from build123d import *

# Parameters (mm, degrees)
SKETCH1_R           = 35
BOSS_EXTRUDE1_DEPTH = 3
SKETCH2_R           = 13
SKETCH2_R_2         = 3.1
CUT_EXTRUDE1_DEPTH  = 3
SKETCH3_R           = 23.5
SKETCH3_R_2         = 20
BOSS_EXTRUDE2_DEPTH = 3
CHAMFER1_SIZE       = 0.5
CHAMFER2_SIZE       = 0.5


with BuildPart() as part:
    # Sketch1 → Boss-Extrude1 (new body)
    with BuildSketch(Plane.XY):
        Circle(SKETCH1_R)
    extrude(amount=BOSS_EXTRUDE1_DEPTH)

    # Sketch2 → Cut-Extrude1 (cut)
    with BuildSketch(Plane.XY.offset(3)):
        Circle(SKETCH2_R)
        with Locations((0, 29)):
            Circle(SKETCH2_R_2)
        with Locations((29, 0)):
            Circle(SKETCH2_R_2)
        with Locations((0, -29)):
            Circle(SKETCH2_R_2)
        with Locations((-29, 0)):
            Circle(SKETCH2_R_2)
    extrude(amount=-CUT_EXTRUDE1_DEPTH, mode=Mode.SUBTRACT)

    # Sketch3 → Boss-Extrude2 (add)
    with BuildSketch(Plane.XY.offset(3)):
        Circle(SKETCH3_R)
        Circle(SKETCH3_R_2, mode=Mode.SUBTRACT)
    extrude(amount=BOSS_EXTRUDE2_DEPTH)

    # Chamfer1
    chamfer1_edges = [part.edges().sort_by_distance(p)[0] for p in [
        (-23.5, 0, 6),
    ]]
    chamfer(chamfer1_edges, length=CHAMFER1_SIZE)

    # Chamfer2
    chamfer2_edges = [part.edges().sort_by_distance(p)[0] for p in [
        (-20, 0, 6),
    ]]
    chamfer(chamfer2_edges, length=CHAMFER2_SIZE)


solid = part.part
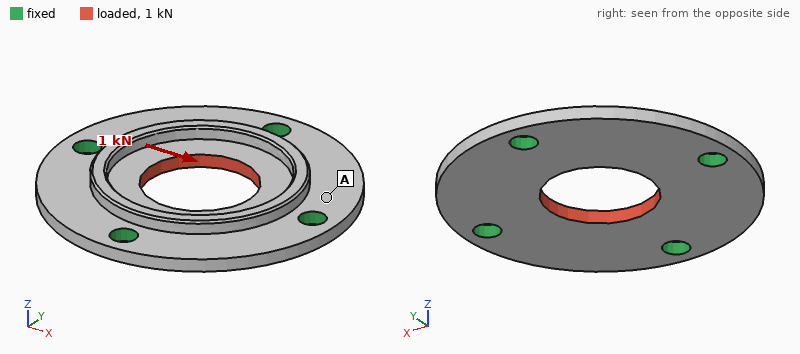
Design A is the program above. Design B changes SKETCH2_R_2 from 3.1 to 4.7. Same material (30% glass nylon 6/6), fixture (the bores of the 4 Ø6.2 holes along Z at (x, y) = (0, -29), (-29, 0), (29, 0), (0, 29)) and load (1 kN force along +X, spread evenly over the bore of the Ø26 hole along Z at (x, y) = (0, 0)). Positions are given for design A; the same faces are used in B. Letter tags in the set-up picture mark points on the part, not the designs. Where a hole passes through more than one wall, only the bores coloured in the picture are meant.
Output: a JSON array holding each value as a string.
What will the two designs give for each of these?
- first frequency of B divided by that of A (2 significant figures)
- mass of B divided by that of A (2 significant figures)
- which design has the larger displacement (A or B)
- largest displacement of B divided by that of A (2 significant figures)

["1.2", "0.96", "A", "0.85"]
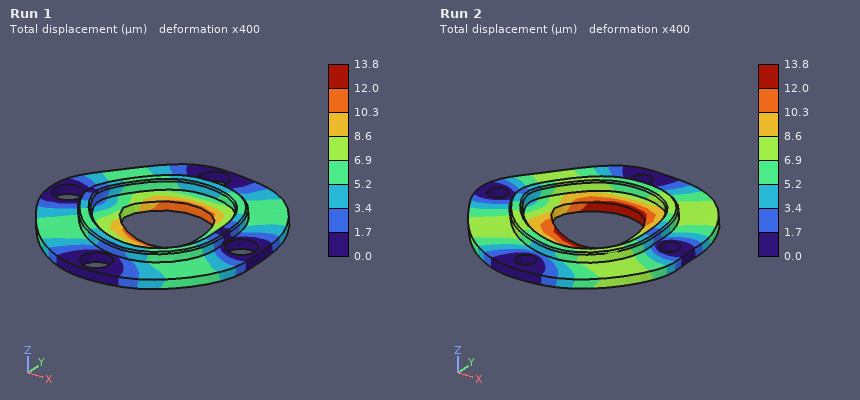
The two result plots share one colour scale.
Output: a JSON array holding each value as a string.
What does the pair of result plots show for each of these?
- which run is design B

["Run 1"]
